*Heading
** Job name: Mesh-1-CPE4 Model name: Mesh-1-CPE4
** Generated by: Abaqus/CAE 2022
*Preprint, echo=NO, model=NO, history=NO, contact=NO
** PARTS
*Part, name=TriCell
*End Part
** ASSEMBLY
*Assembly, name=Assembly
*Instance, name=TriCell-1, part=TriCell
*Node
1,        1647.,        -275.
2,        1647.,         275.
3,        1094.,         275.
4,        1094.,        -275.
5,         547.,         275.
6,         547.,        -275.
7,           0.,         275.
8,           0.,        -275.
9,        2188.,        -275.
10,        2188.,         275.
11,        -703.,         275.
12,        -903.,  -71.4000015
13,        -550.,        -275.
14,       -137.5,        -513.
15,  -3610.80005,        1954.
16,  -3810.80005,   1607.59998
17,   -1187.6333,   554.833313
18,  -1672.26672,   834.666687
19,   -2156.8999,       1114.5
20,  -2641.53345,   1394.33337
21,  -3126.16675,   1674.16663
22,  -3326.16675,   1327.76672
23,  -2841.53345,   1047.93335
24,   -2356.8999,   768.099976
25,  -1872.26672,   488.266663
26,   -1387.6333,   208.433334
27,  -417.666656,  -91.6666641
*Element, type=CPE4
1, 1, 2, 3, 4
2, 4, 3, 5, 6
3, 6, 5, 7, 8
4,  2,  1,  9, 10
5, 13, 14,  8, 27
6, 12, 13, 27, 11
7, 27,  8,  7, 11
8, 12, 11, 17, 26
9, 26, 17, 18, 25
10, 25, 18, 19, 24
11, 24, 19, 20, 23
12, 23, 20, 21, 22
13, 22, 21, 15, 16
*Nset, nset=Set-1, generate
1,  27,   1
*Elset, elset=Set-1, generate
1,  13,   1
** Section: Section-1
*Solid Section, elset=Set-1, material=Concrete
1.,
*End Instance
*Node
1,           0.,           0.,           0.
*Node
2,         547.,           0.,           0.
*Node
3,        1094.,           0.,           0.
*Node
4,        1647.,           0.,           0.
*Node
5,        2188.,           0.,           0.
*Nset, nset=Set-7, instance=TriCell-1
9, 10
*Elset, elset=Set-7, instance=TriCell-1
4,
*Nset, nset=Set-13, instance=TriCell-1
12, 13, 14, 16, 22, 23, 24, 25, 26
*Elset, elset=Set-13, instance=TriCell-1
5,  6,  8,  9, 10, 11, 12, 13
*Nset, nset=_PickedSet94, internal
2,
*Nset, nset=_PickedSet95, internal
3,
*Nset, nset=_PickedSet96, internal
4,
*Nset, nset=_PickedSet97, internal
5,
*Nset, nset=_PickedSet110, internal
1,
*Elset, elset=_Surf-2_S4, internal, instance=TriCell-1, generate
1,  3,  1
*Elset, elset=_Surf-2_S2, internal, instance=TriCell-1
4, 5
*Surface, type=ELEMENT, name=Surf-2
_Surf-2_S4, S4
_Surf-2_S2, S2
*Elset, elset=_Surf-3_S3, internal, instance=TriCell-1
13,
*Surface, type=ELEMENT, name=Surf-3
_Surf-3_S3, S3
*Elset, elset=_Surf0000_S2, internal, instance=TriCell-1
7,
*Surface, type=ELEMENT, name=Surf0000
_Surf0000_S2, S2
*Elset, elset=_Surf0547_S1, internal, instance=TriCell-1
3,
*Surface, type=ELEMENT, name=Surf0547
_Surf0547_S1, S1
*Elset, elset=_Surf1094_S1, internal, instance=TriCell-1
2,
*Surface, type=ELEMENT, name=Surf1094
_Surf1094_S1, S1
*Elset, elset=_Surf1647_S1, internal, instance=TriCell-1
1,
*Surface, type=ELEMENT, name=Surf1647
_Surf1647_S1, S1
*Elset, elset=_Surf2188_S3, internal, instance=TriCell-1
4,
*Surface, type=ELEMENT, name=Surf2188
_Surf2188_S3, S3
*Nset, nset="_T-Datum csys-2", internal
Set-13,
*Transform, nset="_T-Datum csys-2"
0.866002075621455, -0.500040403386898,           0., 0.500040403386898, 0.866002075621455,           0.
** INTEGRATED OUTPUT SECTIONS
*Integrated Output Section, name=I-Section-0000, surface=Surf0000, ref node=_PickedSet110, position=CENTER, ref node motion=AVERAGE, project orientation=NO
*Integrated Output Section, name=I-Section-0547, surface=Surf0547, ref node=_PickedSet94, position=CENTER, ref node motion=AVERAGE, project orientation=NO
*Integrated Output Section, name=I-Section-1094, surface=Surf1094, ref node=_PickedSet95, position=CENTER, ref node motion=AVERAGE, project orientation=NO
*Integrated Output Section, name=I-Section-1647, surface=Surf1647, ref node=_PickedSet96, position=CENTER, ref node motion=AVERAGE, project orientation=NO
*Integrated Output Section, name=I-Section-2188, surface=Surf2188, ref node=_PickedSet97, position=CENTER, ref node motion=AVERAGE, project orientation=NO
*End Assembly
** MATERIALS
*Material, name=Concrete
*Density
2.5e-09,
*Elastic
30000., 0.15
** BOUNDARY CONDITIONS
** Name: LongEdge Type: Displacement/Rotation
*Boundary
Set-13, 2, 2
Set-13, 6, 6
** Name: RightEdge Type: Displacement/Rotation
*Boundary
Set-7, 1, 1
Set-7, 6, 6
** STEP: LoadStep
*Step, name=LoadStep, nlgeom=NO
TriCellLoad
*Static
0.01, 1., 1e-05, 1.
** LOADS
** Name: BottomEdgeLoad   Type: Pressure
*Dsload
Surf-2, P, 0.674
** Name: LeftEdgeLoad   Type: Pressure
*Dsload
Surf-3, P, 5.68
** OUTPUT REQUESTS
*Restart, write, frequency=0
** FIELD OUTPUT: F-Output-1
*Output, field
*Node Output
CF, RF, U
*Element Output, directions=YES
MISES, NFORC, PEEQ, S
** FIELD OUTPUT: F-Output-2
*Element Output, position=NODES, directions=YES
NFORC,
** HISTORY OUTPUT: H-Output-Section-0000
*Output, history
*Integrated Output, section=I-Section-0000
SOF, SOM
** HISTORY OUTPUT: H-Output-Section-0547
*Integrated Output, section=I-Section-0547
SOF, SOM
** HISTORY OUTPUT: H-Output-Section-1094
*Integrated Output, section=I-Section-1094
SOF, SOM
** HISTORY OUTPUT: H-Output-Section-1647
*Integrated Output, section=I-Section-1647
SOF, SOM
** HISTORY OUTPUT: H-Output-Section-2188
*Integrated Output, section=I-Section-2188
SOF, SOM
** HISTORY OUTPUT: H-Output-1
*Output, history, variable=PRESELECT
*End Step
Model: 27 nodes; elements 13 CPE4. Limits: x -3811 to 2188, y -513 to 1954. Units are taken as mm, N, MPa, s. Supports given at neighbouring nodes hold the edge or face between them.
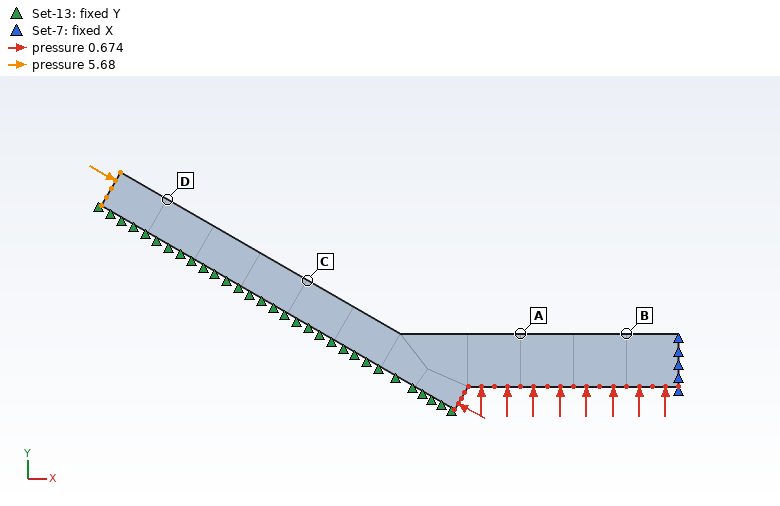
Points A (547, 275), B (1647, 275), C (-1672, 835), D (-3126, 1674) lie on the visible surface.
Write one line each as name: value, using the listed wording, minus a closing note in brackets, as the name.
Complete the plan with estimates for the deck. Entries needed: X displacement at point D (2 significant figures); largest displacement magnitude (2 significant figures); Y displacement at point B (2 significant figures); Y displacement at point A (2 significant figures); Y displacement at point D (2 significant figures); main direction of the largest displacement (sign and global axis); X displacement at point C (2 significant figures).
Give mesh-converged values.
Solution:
X displacement at point D: 0.80 mm
largest displacement magnitude: 2.7 mm
Y displacement at point B: 2.4 mm
Y displacement at point A: 0.81 mm
Y displacement at point D: -0.44 mm
main direction of the largest displacement: +Y
X displacement at point C: 0.53 mm
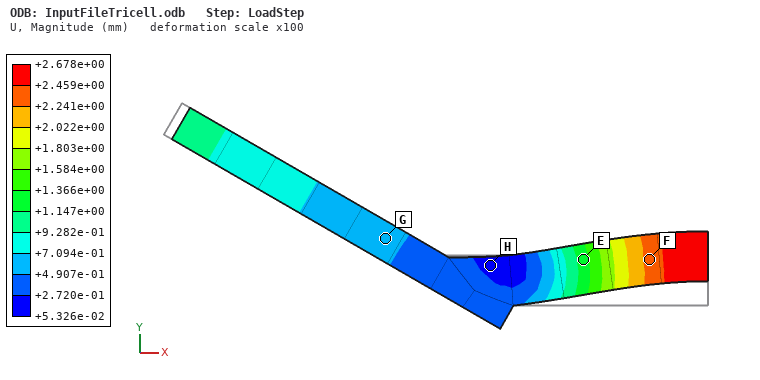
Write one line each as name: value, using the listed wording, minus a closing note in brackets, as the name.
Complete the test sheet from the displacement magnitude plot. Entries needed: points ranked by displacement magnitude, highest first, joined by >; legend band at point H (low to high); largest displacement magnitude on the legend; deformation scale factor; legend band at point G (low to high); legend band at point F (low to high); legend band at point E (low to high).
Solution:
points ranked by displacement magnitude, highest first, joined by >: F > E > G > H
legend band at point H: +5.326e-02 to +2.720e-01 mm
largest displacement magnitude on the legend: +2.678e+00 mm
deformation scale factor: 100
legend band at point G: +4.907e-01 to +7.094e-01 mm
legend band at point F: +2.241e+00 to +2.459e+00 mm
legend band at point E: +1.147e+00 to +1.366e+00 mm
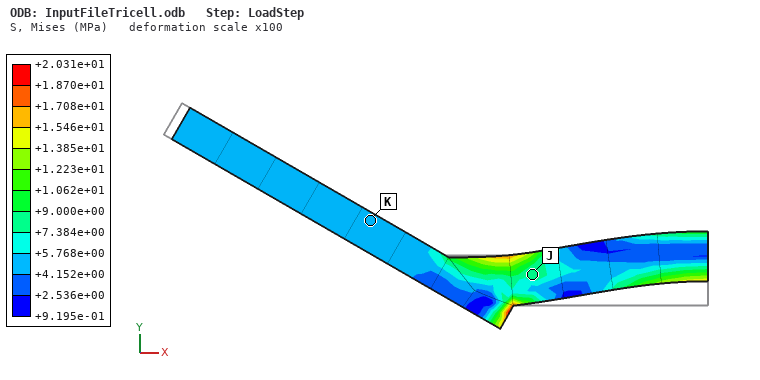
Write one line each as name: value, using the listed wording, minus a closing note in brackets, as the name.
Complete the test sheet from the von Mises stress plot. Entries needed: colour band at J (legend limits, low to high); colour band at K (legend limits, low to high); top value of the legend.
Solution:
colour band at J: +7.384e+00 to +9.000e+00 MPa
colour band at K: +4.152e+00 to +5.768e+00 MPa
top value of the legend: +2.031e+01 MPa
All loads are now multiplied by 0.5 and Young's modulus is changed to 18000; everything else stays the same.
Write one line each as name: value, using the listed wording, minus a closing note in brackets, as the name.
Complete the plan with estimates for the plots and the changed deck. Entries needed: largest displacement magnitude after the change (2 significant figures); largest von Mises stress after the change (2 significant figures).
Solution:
largest displacement magnitude after the change: 2.2 mm
largest von Mises stress after the change: 10 MPa
